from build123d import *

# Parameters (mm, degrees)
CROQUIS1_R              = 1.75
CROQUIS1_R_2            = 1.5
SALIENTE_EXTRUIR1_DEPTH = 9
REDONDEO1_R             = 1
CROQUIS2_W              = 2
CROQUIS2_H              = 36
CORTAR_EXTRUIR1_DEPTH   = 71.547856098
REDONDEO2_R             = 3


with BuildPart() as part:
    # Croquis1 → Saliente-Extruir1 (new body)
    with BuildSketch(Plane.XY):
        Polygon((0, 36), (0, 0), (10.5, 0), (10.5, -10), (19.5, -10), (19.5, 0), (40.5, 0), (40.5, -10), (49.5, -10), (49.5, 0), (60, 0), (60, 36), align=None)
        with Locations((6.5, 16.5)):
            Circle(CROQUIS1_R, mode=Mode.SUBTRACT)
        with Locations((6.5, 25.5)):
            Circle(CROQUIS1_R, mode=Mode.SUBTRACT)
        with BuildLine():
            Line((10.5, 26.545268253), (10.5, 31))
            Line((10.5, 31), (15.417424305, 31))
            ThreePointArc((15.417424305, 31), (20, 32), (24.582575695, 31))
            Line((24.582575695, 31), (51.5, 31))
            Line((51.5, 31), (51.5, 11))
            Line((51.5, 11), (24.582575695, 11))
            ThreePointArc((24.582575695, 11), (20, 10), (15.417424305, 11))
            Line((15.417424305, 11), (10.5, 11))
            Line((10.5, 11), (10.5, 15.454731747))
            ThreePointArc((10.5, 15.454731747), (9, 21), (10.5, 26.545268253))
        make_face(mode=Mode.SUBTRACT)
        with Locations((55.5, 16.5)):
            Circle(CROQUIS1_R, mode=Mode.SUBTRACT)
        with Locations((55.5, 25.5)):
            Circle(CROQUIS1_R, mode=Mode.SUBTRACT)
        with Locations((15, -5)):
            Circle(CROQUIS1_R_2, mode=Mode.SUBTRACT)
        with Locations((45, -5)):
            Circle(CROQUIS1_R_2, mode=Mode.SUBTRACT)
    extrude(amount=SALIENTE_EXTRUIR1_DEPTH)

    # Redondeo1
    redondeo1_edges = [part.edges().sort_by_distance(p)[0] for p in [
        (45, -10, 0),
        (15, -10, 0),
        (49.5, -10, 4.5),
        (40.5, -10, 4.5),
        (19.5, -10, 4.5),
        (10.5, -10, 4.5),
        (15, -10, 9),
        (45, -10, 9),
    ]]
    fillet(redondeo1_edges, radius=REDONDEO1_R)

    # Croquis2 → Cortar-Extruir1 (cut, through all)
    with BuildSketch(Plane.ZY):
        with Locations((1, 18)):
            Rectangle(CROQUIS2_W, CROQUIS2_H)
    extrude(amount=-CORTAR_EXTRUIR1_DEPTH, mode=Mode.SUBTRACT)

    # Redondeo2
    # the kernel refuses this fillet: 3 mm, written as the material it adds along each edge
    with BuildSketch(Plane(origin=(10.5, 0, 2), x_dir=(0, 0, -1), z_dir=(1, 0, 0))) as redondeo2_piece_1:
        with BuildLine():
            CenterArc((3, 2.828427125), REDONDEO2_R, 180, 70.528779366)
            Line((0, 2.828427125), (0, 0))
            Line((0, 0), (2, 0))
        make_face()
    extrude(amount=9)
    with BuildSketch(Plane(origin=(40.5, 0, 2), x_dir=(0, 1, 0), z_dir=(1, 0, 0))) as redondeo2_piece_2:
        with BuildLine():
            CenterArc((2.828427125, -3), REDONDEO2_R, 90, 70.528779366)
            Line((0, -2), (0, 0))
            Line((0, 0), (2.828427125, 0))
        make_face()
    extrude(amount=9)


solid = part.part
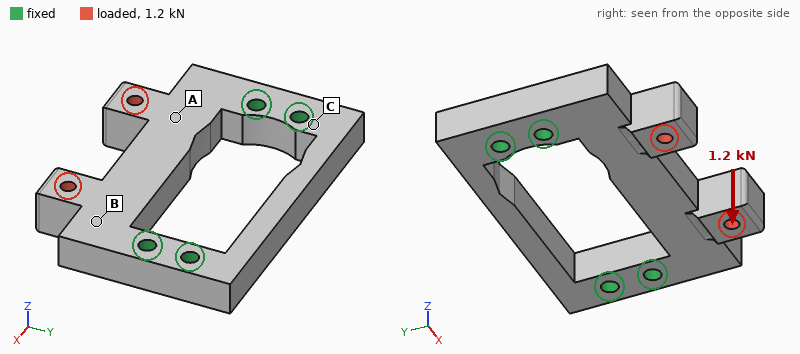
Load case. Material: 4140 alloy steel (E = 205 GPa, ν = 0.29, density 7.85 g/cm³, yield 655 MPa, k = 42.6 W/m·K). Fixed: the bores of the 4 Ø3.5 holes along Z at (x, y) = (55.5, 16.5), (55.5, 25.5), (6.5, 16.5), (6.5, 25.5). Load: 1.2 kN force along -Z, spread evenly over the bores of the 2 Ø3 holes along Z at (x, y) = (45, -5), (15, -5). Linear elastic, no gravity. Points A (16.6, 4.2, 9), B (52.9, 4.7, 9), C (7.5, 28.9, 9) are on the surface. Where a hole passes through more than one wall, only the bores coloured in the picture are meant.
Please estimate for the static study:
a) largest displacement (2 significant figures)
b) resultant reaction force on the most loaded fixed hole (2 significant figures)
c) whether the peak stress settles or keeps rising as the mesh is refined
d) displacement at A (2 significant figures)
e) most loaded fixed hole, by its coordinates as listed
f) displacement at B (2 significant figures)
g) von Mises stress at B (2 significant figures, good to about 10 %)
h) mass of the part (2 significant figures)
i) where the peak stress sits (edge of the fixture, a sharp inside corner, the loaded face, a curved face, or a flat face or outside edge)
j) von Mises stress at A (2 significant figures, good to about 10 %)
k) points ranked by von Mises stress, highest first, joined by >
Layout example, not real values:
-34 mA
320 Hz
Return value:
64 µm
820 N
keeps rising
23 µm
(6.5, 16.5)
17 µm
78 MPa
82 g
edge of the fixture
43 MPa
B > A > C
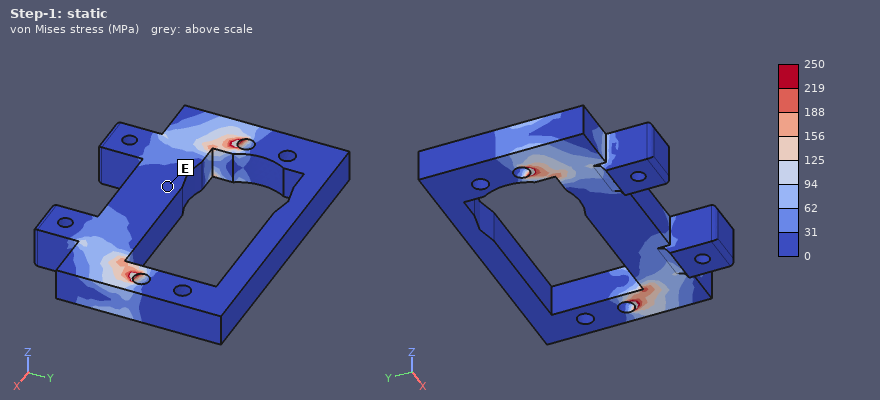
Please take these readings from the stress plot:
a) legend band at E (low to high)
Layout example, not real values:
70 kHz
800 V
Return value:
0 to 31 MPa
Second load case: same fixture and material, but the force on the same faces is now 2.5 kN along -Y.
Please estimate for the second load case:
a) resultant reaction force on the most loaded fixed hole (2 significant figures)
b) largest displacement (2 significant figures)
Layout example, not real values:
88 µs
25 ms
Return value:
1.5 kN
13 µm
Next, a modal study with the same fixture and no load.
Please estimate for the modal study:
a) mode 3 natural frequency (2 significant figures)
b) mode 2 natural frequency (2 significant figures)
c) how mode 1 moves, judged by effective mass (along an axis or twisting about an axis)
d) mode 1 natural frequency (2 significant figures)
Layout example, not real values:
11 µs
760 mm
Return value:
11 kHz
10 kHz
along Z
5800 Hz
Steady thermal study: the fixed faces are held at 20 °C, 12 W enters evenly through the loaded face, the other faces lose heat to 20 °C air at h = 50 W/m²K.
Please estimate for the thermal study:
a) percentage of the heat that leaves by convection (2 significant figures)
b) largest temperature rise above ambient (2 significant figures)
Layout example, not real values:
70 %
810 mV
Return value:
28 %
38 K
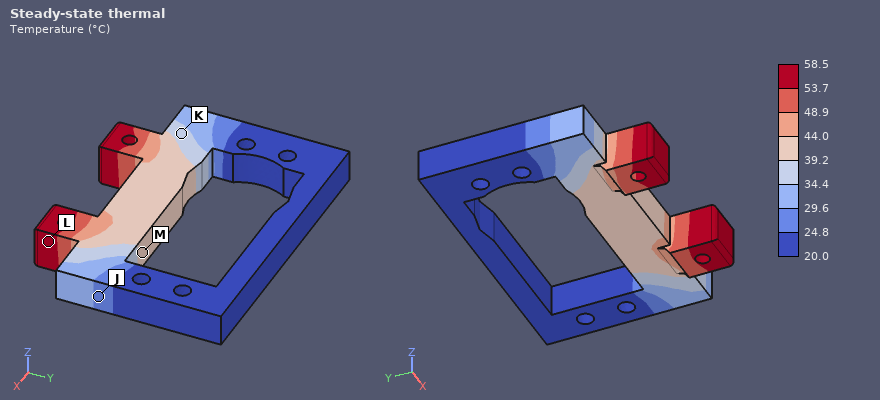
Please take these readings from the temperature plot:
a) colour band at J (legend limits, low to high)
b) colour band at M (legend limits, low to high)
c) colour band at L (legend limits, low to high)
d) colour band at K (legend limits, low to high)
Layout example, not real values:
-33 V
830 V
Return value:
24.8 to 29.6 °C
39.2 to 44.0 °C
53.7 to 58.5 °C
34.4 to 39.2 °C
